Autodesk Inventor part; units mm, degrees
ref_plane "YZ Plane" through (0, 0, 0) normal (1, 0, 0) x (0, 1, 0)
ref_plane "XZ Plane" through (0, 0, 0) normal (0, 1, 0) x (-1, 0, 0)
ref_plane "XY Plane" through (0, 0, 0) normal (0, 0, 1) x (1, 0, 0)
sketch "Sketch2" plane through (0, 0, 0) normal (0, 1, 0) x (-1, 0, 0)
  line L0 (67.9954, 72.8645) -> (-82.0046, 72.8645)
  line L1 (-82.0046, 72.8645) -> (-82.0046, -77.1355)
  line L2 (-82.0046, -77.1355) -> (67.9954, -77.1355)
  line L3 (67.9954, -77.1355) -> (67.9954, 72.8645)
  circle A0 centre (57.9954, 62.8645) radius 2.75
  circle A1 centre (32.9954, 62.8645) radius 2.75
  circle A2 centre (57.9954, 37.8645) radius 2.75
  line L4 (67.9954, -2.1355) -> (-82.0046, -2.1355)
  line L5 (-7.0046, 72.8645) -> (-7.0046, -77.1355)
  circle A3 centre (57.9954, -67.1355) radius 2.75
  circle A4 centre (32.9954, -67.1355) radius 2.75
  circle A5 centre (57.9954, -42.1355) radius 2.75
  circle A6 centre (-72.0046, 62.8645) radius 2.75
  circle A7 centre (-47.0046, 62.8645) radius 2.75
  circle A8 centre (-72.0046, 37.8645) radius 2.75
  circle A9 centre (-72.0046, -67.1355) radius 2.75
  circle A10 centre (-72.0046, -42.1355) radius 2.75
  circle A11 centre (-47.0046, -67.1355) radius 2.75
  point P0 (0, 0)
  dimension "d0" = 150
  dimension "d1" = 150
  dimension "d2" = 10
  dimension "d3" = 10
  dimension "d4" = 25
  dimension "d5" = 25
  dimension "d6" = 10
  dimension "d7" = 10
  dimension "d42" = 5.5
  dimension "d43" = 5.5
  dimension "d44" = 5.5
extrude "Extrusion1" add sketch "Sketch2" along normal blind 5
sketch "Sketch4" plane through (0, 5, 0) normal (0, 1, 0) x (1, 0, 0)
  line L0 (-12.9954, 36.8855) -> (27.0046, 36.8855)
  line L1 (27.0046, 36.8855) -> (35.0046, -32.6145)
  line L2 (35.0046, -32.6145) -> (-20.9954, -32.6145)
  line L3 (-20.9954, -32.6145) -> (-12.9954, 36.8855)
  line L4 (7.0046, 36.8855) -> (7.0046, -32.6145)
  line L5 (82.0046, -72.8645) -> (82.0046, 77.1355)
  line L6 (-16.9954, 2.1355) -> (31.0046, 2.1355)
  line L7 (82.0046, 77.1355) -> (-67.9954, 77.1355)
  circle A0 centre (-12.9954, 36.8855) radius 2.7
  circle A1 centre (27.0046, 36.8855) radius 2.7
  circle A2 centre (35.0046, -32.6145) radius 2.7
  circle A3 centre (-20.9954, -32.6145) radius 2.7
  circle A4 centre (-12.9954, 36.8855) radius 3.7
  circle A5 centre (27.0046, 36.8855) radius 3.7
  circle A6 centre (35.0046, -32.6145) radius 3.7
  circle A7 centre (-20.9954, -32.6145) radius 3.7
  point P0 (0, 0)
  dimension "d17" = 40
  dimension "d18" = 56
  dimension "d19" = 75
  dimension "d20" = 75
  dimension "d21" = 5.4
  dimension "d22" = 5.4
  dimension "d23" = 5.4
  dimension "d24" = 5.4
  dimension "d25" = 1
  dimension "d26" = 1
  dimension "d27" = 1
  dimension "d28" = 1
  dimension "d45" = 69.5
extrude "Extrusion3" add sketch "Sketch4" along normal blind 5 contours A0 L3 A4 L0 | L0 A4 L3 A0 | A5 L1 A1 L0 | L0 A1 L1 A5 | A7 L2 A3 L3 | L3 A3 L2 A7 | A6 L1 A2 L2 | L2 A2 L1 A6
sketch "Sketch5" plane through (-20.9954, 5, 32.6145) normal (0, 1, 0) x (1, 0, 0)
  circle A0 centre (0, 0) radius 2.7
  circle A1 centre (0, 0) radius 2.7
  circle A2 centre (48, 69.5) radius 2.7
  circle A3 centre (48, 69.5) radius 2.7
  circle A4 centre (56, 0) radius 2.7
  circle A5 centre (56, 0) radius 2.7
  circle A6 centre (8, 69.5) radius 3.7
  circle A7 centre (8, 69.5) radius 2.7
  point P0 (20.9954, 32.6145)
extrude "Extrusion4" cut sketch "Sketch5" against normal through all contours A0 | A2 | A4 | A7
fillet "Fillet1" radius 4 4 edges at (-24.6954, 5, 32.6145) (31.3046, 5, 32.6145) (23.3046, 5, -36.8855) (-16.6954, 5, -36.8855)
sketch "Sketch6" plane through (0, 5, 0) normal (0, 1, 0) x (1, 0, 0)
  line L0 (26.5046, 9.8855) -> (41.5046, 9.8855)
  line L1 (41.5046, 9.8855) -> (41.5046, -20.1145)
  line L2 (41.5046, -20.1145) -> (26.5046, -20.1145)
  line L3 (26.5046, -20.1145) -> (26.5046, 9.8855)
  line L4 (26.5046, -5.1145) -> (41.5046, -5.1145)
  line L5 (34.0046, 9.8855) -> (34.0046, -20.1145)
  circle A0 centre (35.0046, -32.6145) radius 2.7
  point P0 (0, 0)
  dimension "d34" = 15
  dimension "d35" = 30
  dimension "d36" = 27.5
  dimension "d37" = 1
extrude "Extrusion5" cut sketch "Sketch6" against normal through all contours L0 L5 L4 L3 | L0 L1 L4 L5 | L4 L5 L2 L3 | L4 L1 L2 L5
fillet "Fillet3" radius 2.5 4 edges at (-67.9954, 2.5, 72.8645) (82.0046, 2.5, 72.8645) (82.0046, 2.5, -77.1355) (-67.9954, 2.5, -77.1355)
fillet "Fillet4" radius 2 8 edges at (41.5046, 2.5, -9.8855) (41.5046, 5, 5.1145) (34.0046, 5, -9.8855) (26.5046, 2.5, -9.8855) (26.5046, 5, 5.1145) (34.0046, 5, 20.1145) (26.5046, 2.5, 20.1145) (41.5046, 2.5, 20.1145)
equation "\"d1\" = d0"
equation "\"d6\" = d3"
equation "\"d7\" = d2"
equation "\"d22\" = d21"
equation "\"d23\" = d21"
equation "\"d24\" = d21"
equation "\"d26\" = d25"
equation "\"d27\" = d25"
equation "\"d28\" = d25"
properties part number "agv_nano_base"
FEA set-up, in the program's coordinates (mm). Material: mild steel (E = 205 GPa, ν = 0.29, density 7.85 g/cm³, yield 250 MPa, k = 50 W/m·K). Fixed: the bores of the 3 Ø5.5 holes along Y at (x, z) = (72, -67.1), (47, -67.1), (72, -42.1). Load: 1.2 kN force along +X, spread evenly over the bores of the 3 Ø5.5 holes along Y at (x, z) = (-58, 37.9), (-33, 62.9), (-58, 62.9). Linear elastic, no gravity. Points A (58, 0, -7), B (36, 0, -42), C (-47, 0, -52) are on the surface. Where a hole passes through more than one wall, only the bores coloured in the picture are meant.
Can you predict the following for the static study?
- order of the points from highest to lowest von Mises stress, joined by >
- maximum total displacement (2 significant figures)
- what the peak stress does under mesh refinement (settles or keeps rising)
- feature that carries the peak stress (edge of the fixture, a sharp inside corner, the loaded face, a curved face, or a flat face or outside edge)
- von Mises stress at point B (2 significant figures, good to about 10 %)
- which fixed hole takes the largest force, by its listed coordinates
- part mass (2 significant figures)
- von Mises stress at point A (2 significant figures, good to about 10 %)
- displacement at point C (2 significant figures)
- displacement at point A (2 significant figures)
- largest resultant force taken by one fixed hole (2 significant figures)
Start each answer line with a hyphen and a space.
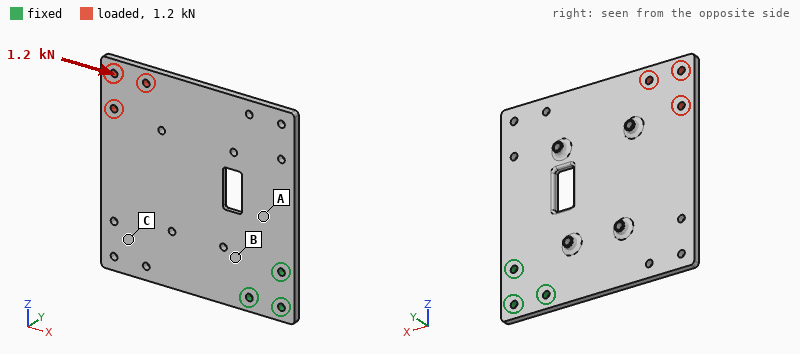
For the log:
- B > A > C
- 49 µm
- keeps rising
- edge of the fixture
- 16 MPa
- (72, -42.1)
- 860 g
- 9.2 MPa
- 27 µm
- 11 µm
- 3.6 kN
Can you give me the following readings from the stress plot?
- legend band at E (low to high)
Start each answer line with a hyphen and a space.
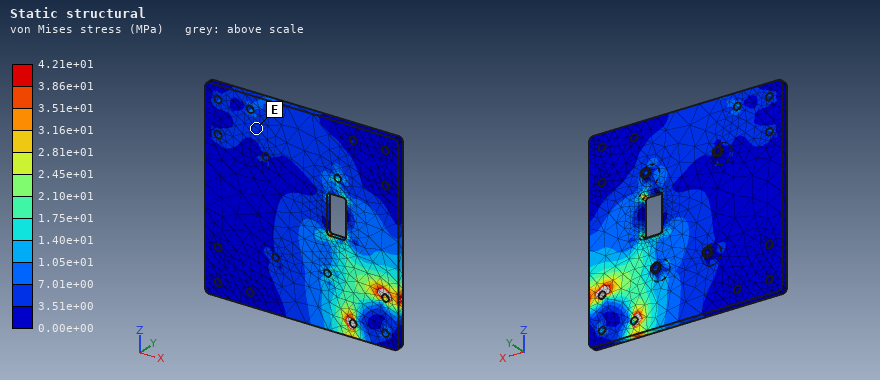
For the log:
- 3.51e+00 to 7.01e+00 MPa
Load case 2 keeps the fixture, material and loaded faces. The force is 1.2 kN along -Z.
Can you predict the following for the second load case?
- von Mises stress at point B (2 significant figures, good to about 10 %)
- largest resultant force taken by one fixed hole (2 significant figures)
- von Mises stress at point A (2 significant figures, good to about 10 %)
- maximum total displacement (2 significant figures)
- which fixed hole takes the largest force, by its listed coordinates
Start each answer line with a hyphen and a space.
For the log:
- 18 MPa
- 3.6 kN
- 5.6 MPa
- 48 µm
- (47, -67.1)
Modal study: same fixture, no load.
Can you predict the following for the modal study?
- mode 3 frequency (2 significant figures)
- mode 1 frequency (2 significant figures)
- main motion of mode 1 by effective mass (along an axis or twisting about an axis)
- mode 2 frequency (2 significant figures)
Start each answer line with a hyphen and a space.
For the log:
- 670 Hz
- 150 Hz
- along Y
- 320 Hz
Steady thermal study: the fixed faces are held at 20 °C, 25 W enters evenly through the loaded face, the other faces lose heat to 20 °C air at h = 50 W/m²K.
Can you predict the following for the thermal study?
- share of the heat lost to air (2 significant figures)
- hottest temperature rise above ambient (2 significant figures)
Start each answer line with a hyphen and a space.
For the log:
- 96 %
- 61 K
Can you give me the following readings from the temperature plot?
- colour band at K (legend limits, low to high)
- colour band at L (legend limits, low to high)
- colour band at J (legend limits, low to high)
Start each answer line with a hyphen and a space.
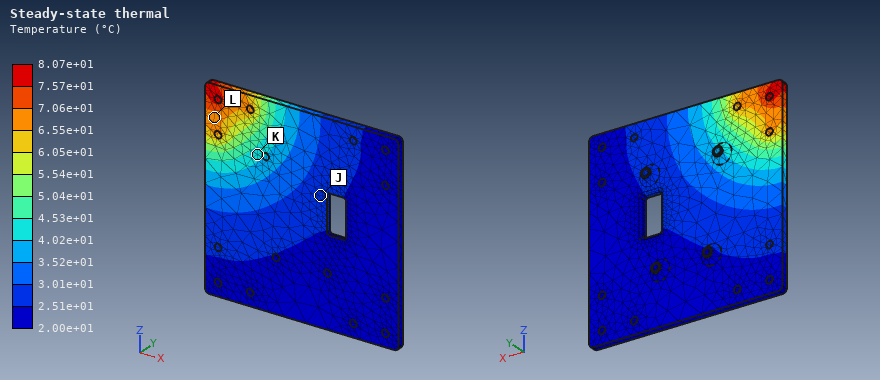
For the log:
- 4.02e+01 to 4.53e+01 °C
- 6.55e+01 to 7.06e+01 °C
- 2.51e+01 to 3.01e+01 °C
